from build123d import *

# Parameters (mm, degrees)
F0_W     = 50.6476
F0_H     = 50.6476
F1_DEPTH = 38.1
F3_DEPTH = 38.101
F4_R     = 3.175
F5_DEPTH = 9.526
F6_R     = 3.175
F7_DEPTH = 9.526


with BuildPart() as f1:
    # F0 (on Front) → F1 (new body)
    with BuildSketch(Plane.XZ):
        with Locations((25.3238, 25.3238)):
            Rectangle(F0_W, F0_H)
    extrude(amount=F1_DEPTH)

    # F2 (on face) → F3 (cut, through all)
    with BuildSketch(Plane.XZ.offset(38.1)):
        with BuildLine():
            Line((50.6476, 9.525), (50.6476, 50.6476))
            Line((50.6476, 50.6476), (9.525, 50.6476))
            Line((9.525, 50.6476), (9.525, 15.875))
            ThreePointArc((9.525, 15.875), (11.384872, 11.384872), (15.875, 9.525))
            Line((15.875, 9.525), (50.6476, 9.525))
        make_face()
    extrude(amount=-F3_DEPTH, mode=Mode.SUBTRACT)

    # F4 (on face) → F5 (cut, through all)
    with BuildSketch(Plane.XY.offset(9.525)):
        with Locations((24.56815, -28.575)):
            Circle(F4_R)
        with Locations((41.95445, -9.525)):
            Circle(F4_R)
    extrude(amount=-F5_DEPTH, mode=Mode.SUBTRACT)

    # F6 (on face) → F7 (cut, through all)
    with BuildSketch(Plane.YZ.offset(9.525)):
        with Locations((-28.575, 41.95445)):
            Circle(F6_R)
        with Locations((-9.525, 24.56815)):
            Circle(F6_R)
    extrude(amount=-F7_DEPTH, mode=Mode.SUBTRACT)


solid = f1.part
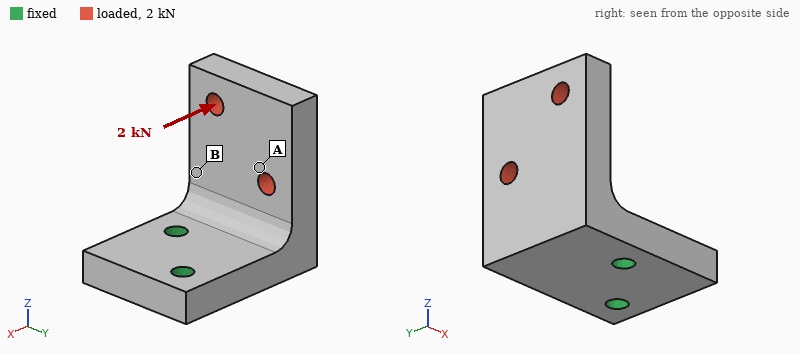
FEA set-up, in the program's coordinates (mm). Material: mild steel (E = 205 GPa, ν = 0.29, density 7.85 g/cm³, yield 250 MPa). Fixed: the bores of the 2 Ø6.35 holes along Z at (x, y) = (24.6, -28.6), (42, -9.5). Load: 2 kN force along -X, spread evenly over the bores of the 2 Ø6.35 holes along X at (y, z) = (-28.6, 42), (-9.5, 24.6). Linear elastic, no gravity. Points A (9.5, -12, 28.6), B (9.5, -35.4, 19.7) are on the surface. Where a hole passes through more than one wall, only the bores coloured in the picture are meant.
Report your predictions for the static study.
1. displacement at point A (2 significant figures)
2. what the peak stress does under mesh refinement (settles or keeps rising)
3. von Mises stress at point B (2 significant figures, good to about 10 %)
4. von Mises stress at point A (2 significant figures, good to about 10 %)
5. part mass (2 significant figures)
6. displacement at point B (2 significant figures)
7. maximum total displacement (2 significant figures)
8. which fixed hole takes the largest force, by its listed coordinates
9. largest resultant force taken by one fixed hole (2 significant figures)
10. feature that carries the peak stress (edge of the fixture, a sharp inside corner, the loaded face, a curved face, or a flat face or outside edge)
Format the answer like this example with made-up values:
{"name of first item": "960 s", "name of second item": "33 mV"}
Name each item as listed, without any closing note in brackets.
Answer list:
{"displacement at point A": "0.056 mm", "what the peak stress does under mesh refinement": "keeps rising", "von Mises stress at point B": "57 MPa", "von Mises stress at point A": "20 MPa", "part mass": "250 g", "displacement at point B": "0.031 mm", "maximum total displacement": "0.13 mm", "which fixed hole takes the largest force, by its listed coordinates": "(24.6, -28.6)", "largest resultant force taken by one fixed hole": "1.4 kN", "feature that carries the peak stress": "edge of the fixture"}
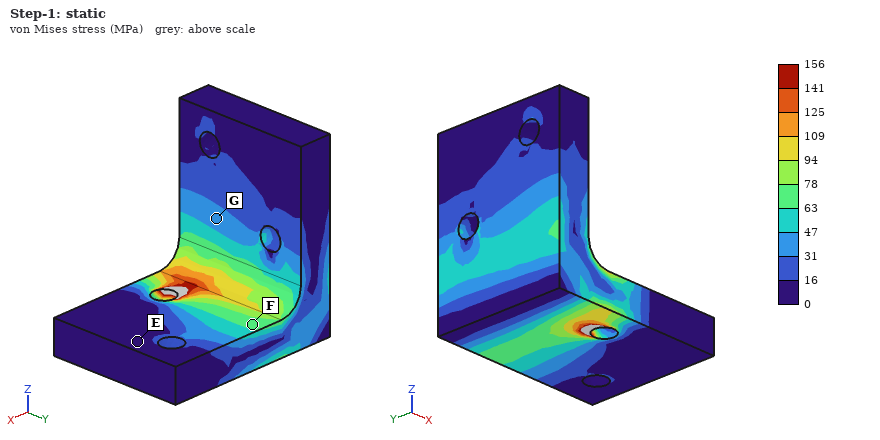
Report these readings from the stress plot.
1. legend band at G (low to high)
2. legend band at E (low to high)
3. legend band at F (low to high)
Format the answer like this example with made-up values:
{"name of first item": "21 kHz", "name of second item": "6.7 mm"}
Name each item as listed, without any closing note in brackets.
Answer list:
{"legend band at G": "31 to 47 MPa", "legend band at E": "0 to 16 MPa", "legend band at F": "63 to 78 MPa"}
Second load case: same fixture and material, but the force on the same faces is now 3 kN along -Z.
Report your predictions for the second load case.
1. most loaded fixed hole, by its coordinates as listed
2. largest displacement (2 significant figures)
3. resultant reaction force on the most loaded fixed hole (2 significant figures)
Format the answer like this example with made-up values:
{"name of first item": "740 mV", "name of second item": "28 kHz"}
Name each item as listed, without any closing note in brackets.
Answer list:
{"most loaded fixed hole, by its coordinates as listed": "(24.6, -28.6)", "largest displacement": "75 µm", "resultant reaction force on the most loaded fixed hole": "3.1 kN"}
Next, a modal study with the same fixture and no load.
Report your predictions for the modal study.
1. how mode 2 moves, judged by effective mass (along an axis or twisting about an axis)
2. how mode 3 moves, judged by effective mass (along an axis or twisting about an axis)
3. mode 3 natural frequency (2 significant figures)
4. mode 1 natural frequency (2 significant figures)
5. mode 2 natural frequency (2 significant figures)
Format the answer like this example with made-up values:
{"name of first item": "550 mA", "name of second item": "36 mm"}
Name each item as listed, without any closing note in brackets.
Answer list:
{"how mode 2 moves, judged by effective mass": "along Y", "how mode 3 moves, judged by effective mass": "along Z", "mode 3 natural frequency": "7500 Hz", "mode 1 natural frequency": "2300 Hz", "mode 2 natural frequency": "3400 Hz"}
